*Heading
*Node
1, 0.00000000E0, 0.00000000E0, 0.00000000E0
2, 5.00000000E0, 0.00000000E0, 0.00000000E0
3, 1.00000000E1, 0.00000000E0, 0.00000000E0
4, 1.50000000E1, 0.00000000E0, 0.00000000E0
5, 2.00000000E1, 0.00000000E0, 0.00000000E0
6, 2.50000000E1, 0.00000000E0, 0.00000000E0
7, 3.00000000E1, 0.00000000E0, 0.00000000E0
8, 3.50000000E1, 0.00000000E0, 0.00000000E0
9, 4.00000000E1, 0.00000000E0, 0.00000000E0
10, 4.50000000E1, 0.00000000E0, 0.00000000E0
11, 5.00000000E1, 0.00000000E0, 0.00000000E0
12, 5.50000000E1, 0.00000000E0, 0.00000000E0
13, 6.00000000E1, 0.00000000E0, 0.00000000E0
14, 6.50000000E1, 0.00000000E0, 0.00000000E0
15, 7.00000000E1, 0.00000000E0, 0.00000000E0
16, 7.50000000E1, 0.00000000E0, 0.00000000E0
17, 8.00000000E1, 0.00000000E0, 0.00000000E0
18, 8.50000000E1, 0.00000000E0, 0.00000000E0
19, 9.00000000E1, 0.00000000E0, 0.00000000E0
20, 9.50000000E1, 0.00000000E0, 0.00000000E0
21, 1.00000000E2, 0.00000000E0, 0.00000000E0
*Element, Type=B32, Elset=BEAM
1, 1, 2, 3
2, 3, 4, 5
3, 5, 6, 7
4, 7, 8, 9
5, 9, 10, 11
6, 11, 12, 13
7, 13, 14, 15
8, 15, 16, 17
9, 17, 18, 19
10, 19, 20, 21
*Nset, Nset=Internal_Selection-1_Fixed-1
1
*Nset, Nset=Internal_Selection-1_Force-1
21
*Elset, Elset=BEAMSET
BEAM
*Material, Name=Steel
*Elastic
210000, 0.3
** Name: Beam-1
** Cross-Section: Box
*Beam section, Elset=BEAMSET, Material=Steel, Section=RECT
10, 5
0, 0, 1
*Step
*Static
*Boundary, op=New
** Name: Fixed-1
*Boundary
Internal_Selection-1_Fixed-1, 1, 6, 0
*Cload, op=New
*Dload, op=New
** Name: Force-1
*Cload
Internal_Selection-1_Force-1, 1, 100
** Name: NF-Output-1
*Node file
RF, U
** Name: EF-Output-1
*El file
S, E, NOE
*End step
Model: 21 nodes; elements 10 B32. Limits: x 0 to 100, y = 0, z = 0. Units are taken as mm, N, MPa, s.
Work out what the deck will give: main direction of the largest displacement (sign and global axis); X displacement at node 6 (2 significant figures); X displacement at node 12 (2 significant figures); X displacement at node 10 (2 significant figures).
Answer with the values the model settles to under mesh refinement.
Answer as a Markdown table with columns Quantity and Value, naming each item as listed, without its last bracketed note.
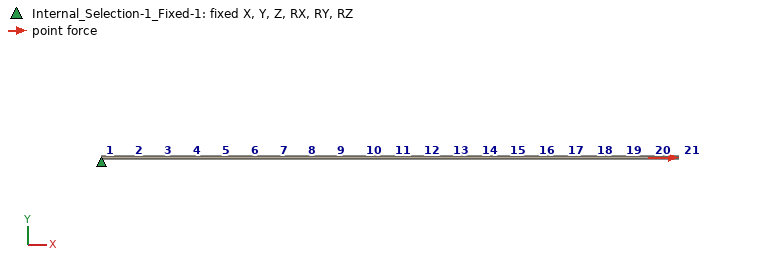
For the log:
| Quantity | Value |
|---|---|
| main direction of the largest displacement | +X |
| X displacement at node 6 | 2.4e-04 mm |
| X displacement at node 12 | 5.2e-04 mm |
| X displacement at node 10 | 4.3e-04 mm |
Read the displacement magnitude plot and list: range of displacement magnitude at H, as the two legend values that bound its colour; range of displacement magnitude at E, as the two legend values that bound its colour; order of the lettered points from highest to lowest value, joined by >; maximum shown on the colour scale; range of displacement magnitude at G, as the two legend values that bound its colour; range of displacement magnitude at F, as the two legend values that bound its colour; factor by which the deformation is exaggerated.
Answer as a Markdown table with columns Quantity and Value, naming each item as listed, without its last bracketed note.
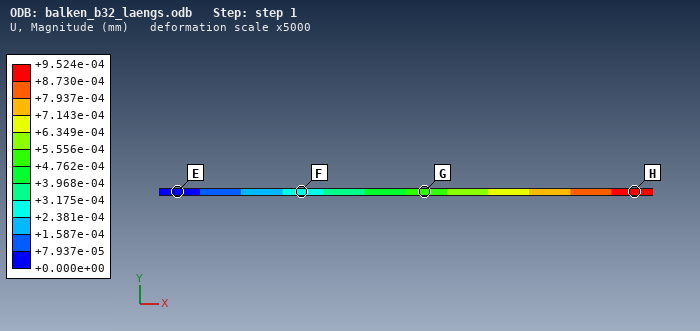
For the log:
| Quantity | Value |
|---|---|
| range of displacement magnitude at H, as the two legend values that bound its colour | +8.730e-04 to +9.524e-04 mm |
| range of displacement magnitude at E, as the two legend values that bound its colour | +0.000e+00 to +7.937e-05 mm |
| order of the lettered points from highest to lowest value, joined by > | H > G > F > E |
| maximum shown on the colour scale | +9.524e-04 mm |
| range of displacement magnitude at G, as the two legend values that bound its colour | +4.762e-04 to +5.556e-04 mm |
| range of displacement magnitude at F, as the two legend values that bound its colour | +2.381e-04 to +3.175e-04 mm |
| factor by which the deformation is exaggerated | 5000 |
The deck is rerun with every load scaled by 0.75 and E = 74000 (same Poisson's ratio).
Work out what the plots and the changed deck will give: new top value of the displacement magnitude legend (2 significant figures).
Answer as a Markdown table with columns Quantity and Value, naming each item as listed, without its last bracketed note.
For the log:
| Quantity | Value |
|---|---|
| new top value of the displacement magnitude legend | 0.0020 mm |
